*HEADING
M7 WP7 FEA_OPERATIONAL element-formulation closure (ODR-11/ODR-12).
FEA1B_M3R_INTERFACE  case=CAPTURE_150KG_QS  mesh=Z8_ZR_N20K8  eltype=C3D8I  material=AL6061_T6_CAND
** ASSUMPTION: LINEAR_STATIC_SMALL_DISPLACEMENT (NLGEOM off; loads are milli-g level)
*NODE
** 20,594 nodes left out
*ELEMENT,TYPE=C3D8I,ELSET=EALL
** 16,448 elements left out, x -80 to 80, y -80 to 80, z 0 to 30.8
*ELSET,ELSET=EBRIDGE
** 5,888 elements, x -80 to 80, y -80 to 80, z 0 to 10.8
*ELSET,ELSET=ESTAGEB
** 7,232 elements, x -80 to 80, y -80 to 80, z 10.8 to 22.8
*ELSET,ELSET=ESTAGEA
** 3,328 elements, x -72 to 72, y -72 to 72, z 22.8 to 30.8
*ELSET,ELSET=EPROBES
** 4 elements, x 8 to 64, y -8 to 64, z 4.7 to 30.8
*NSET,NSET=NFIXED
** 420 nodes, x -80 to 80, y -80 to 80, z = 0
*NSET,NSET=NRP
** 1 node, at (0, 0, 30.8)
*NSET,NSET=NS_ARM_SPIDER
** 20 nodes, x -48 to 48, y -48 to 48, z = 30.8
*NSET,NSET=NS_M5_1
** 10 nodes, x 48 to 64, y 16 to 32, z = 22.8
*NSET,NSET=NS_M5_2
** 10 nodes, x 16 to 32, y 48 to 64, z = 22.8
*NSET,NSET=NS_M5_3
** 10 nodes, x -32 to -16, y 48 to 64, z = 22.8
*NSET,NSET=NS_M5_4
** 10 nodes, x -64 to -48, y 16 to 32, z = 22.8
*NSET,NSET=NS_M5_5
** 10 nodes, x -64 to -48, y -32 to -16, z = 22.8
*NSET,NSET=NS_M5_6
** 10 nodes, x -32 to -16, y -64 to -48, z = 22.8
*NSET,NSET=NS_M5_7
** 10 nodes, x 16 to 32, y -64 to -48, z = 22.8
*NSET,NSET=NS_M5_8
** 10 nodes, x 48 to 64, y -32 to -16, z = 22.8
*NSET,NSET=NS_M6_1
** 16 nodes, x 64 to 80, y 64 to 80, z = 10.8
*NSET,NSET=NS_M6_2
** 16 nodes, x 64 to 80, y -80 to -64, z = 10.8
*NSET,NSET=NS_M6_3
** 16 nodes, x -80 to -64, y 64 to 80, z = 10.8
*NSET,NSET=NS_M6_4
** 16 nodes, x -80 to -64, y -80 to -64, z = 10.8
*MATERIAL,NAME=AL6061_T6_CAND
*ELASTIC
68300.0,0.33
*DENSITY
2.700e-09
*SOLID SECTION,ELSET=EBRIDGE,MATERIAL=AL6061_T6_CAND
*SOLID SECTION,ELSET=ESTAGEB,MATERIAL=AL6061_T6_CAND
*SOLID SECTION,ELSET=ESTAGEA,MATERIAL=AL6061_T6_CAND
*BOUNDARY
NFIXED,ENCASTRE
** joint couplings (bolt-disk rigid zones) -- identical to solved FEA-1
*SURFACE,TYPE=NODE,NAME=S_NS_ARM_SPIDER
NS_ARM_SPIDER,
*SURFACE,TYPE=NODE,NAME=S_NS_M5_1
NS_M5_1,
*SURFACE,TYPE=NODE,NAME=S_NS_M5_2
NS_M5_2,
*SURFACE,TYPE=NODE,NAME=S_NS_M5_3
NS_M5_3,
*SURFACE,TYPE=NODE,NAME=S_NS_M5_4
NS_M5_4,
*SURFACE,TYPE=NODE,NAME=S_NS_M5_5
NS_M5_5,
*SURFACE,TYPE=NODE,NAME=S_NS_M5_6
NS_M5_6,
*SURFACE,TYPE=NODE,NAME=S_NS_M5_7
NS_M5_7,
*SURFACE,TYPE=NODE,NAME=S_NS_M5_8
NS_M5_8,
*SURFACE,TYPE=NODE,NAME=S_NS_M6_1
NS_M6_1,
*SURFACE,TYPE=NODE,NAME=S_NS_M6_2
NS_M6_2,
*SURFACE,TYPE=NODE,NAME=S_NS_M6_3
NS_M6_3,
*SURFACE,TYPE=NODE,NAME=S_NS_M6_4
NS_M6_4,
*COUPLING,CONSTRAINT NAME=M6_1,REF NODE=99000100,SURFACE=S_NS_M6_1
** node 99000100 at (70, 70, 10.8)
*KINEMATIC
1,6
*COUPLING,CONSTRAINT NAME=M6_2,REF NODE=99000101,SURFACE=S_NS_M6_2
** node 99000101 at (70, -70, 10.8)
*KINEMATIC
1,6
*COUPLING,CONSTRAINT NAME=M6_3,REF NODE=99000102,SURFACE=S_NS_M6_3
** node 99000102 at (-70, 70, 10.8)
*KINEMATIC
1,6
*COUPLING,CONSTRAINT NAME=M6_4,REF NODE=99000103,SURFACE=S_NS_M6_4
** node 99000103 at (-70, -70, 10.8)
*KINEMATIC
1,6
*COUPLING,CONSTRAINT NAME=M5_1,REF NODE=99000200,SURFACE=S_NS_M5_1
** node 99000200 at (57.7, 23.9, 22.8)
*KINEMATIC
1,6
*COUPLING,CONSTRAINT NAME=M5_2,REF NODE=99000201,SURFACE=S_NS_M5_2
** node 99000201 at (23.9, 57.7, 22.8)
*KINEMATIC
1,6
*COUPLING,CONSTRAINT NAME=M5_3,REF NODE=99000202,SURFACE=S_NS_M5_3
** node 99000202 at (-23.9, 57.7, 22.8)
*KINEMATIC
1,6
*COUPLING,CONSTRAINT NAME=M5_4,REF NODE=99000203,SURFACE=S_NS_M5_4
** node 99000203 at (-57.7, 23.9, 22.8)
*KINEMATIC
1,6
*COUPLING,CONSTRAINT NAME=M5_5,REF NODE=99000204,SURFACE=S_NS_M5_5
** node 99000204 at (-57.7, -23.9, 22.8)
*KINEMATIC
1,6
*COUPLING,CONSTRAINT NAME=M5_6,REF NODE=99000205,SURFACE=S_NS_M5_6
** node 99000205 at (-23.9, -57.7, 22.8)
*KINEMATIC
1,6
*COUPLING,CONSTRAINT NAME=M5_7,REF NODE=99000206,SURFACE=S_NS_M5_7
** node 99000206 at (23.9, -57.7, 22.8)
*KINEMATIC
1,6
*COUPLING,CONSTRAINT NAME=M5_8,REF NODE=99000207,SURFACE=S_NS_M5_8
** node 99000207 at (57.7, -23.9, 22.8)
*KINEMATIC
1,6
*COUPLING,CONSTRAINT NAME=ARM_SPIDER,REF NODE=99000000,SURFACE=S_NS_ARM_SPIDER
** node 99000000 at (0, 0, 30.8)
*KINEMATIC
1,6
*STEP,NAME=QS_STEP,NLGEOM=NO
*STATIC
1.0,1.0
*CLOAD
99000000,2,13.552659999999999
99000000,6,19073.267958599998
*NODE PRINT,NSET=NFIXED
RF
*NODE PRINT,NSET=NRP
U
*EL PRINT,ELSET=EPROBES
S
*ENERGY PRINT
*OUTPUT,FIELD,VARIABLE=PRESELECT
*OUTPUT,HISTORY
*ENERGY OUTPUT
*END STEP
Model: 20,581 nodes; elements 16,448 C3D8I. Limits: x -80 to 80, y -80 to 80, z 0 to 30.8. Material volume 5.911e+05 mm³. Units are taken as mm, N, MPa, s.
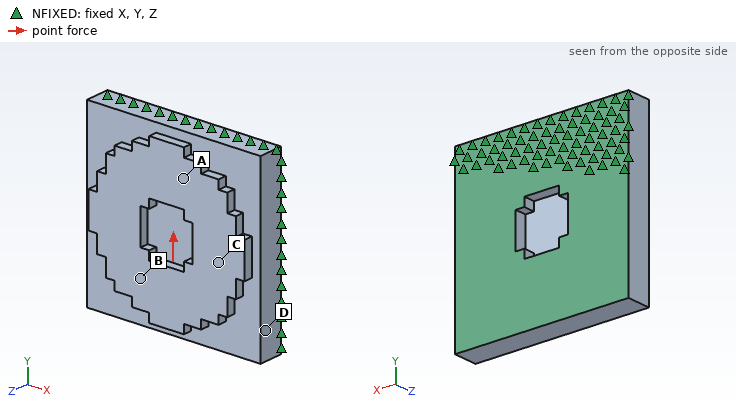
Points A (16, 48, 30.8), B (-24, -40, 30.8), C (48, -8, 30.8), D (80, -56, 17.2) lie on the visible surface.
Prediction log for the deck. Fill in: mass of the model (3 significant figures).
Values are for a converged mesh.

1.60 kg
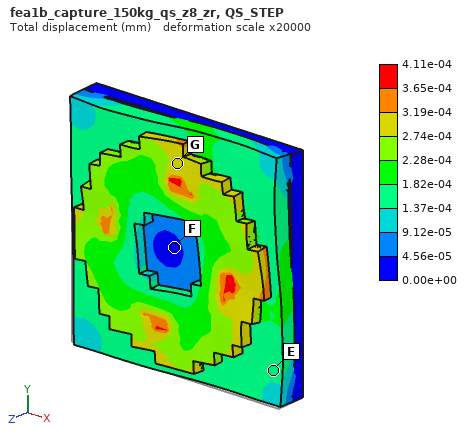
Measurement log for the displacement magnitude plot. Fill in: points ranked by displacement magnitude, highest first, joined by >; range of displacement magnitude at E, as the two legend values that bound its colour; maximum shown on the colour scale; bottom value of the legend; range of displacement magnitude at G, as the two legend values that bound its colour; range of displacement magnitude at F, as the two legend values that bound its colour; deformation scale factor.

G > E > F
1.37e-04 to 1.82e-04 mm
4.11e-04 mm
0.00e+00 mm
2.74e-04 to 3.19e-04 mm
0.00e+00 to 4.56e-05 mm
20000
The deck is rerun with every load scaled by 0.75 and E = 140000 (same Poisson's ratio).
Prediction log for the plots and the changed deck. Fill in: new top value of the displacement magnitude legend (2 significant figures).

1.5e-04 mm
